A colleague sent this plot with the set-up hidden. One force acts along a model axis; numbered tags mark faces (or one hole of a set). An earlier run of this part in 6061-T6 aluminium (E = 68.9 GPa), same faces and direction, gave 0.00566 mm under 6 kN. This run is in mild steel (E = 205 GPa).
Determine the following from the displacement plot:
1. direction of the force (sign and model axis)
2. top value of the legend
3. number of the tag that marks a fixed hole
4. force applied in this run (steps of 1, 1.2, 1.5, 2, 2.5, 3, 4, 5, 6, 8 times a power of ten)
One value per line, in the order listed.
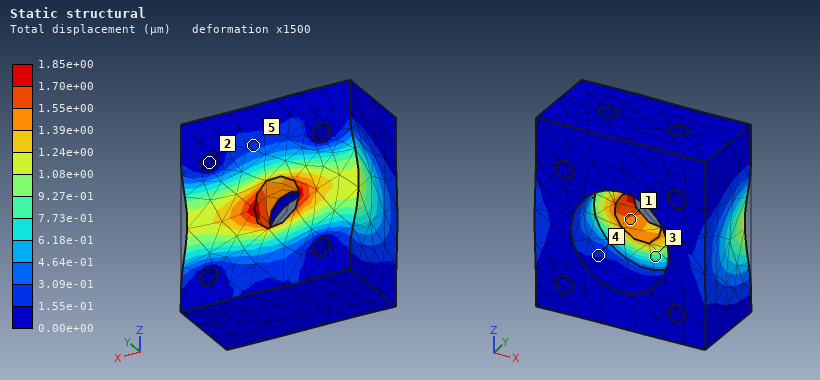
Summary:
-X
1.85e+00 µm
2
6 kN
